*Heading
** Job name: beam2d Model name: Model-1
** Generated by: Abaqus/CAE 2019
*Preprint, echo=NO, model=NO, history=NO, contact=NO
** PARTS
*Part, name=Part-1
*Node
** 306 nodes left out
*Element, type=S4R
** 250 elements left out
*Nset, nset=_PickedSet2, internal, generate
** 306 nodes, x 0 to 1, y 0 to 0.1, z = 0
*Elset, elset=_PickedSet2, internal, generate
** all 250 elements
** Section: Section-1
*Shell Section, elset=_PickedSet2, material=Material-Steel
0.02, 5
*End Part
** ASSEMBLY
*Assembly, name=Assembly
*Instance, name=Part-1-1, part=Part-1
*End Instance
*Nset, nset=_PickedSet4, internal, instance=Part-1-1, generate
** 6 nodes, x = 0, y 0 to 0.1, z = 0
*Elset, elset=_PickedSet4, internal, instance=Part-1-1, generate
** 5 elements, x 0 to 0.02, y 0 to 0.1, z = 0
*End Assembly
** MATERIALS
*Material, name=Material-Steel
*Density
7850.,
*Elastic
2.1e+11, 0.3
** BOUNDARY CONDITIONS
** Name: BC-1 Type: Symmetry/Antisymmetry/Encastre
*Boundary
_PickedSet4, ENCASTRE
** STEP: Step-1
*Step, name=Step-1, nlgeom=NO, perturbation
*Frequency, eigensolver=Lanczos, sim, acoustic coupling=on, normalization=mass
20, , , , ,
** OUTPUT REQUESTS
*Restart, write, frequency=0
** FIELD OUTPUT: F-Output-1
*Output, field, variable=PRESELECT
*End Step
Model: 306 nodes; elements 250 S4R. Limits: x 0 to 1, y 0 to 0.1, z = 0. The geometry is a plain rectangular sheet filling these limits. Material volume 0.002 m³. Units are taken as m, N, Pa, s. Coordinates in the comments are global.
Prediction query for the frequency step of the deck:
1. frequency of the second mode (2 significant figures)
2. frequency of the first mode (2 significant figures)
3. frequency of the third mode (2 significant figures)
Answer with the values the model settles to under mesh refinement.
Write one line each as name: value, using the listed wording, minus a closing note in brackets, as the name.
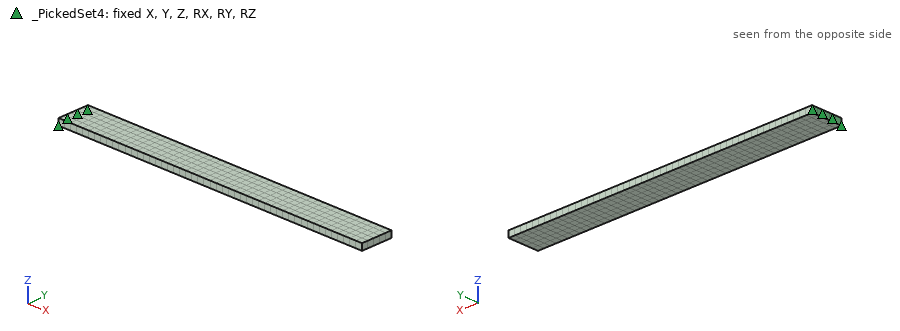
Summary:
frequency of the second mode: 83 Hz
frequency of the first mode: 17 Hz
frequency of the third mode: 110 Hz
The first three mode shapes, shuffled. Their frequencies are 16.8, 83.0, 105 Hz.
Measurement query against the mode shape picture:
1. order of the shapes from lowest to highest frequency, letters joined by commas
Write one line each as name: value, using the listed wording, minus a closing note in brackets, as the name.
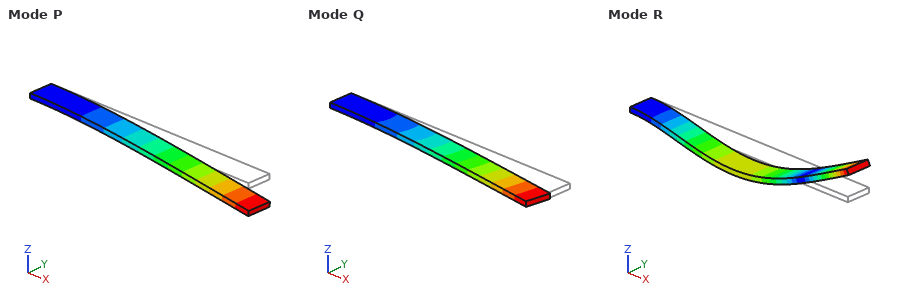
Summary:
order of the shapes from lowest to highest frequency, letters joined by commas: P, Q, R
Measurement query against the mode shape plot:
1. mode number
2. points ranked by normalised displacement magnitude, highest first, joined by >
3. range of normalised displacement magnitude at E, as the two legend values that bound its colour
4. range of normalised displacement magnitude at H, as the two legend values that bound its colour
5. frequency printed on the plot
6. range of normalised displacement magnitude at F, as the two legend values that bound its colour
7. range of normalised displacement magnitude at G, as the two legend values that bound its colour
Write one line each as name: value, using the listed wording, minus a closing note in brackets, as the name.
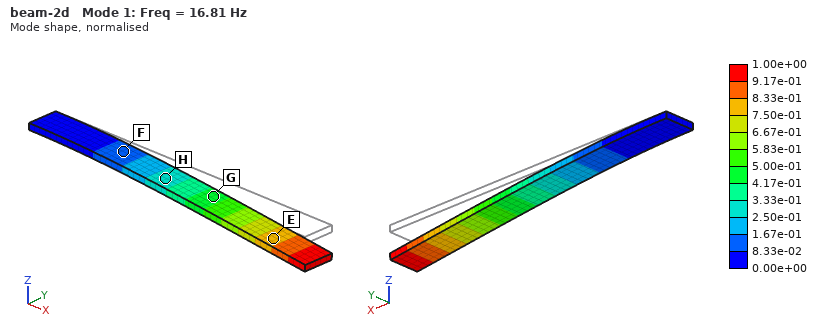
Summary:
mode number: 1
points ranked by normalised displacement magnitude, highest first, joined by >: E > G > H > F
range of normalised displacement magnitude at E, as the two legend values that bound its colour: 7.50e-01 to 8.33e-01
range of normalised displacement magnitude at H, as the two legend values that bound its colour: 2.50e-01 to 3.33e-01
frequency printed on the plot: 16.81 Hz
range of normalised displacement magnitude at F, as the two legend values that bound its colour: 8.33e-02 to 1.67e-01
range of normalised displacement magnitude at G, as the two legend values that bound its colour: 4.17e-01 to 5.00e-01
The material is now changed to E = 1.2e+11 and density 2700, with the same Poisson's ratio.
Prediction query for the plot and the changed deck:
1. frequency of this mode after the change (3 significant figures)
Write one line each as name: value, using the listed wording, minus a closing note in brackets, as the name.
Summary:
frequency of this mode after the change: 21.7 Hz
